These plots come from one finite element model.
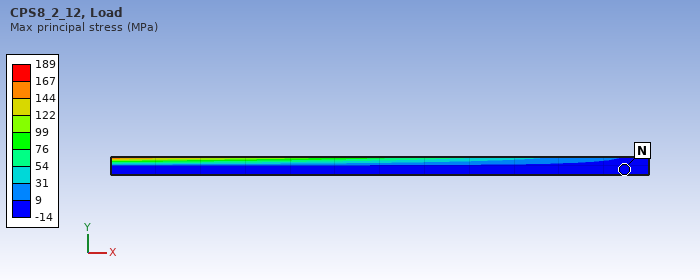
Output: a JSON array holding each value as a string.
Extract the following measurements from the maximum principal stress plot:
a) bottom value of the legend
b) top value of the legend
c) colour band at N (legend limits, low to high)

["-14 MPa", "189 MPa", "-14 to 9 MPa"]
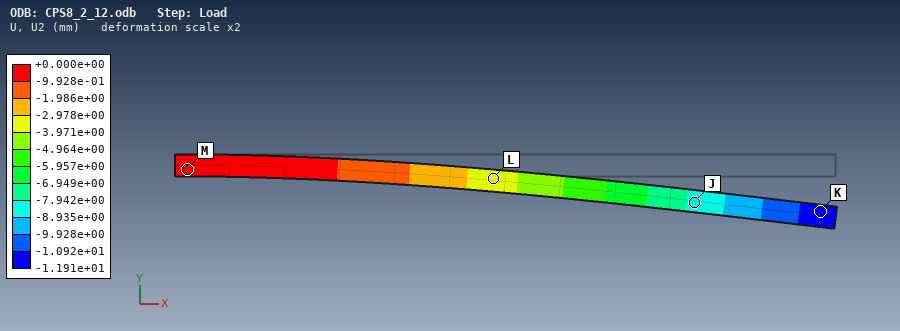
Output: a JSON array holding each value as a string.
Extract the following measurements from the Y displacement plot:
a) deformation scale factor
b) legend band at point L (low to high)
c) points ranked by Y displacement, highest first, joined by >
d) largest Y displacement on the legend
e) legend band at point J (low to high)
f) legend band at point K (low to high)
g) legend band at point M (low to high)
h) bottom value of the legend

["2", "-3.971e+00 to -2.978e+00 mm", "M > L > J > K", "+0.000e+00 mm", "-8.935e+00 to -7.942e+00 mm", "-1.191e+01 to -1.092e+01 mm", "-9.928e-01 to +0.000e+00 mm", "-1.191e+01 mm"]
